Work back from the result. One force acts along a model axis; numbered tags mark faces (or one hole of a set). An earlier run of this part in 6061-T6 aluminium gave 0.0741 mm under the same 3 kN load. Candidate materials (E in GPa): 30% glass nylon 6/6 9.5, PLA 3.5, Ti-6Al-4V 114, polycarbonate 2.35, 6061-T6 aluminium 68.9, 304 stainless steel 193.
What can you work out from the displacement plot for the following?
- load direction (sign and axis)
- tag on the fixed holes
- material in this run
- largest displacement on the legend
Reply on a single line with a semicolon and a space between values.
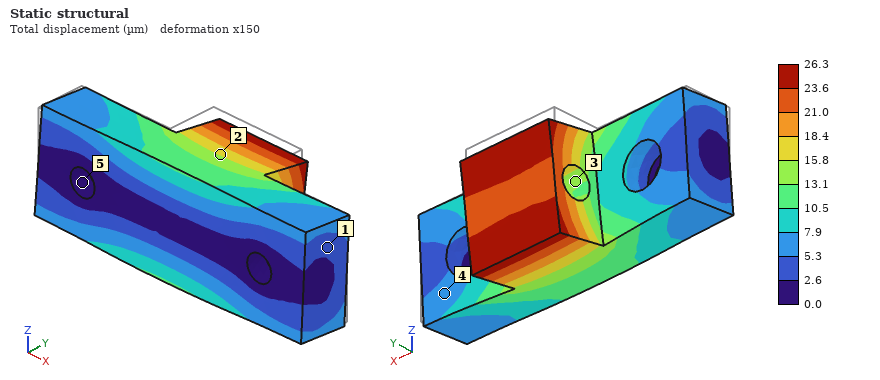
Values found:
-Z; 5; 304 stainless steel; 26.3 µm
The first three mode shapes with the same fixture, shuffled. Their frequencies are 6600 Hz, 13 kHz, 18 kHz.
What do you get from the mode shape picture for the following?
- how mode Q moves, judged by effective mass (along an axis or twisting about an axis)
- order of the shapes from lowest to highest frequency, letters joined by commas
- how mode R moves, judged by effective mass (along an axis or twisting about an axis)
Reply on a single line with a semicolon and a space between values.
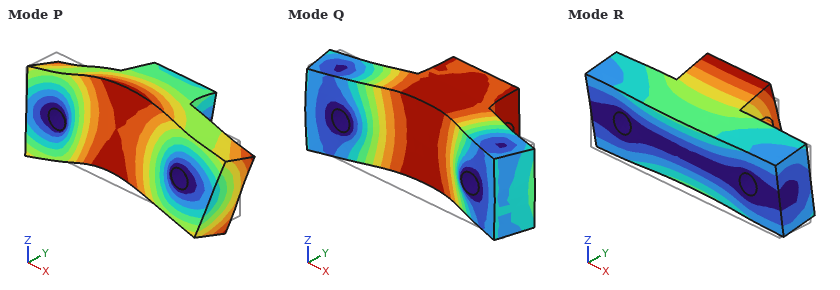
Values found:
along Y; R, Q, P; along Z
